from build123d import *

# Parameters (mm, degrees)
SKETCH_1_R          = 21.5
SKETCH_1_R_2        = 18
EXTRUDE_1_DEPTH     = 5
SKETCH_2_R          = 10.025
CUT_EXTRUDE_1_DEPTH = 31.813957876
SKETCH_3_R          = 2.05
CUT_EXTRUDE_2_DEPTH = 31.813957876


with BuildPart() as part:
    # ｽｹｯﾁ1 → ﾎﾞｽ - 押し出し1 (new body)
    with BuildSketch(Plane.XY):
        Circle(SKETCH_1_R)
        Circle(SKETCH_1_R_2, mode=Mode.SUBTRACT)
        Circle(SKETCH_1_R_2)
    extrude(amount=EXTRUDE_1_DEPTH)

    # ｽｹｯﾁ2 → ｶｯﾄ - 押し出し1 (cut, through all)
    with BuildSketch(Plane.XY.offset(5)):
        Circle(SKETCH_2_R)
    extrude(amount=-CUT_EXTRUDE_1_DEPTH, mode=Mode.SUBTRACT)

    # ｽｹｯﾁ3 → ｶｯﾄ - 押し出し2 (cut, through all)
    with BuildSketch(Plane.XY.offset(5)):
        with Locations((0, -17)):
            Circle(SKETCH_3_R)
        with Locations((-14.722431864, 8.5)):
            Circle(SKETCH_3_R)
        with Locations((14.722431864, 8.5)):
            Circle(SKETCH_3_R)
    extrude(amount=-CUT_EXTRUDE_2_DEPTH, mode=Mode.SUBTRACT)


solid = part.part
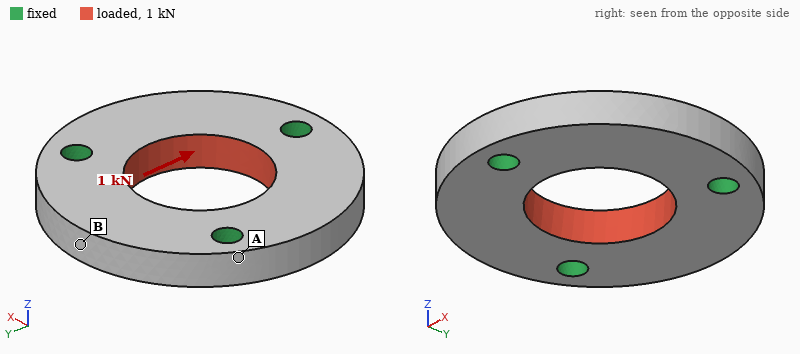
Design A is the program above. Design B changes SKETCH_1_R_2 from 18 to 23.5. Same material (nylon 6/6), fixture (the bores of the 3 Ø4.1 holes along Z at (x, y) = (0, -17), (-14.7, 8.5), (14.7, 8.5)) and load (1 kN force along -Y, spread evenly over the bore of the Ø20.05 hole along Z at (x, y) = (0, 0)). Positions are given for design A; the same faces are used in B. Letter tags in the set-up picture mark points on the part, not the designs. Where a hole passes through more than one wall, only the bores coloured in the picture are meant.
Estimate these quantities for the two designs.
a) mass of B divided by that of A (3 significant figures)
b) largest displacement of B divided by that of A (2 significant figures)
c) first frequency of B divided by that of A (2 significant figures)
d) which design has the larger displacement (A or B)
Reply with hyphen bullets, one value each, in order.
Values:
- 1.26
- 0.87
- 0.86
- A
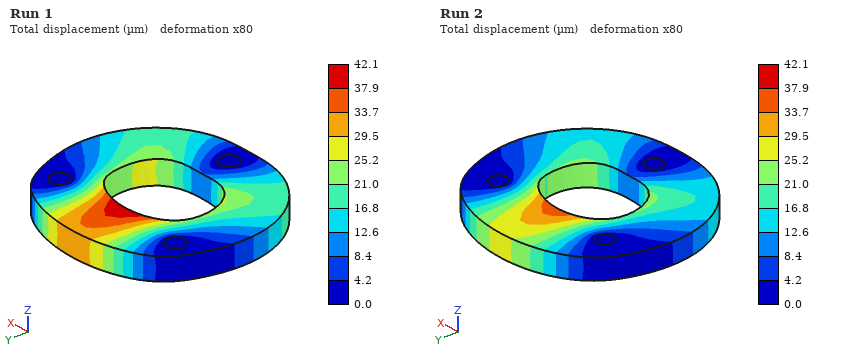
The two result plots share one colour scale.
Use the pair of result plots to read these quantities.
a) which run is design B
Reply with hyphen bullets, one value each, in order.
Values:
- Run 2
